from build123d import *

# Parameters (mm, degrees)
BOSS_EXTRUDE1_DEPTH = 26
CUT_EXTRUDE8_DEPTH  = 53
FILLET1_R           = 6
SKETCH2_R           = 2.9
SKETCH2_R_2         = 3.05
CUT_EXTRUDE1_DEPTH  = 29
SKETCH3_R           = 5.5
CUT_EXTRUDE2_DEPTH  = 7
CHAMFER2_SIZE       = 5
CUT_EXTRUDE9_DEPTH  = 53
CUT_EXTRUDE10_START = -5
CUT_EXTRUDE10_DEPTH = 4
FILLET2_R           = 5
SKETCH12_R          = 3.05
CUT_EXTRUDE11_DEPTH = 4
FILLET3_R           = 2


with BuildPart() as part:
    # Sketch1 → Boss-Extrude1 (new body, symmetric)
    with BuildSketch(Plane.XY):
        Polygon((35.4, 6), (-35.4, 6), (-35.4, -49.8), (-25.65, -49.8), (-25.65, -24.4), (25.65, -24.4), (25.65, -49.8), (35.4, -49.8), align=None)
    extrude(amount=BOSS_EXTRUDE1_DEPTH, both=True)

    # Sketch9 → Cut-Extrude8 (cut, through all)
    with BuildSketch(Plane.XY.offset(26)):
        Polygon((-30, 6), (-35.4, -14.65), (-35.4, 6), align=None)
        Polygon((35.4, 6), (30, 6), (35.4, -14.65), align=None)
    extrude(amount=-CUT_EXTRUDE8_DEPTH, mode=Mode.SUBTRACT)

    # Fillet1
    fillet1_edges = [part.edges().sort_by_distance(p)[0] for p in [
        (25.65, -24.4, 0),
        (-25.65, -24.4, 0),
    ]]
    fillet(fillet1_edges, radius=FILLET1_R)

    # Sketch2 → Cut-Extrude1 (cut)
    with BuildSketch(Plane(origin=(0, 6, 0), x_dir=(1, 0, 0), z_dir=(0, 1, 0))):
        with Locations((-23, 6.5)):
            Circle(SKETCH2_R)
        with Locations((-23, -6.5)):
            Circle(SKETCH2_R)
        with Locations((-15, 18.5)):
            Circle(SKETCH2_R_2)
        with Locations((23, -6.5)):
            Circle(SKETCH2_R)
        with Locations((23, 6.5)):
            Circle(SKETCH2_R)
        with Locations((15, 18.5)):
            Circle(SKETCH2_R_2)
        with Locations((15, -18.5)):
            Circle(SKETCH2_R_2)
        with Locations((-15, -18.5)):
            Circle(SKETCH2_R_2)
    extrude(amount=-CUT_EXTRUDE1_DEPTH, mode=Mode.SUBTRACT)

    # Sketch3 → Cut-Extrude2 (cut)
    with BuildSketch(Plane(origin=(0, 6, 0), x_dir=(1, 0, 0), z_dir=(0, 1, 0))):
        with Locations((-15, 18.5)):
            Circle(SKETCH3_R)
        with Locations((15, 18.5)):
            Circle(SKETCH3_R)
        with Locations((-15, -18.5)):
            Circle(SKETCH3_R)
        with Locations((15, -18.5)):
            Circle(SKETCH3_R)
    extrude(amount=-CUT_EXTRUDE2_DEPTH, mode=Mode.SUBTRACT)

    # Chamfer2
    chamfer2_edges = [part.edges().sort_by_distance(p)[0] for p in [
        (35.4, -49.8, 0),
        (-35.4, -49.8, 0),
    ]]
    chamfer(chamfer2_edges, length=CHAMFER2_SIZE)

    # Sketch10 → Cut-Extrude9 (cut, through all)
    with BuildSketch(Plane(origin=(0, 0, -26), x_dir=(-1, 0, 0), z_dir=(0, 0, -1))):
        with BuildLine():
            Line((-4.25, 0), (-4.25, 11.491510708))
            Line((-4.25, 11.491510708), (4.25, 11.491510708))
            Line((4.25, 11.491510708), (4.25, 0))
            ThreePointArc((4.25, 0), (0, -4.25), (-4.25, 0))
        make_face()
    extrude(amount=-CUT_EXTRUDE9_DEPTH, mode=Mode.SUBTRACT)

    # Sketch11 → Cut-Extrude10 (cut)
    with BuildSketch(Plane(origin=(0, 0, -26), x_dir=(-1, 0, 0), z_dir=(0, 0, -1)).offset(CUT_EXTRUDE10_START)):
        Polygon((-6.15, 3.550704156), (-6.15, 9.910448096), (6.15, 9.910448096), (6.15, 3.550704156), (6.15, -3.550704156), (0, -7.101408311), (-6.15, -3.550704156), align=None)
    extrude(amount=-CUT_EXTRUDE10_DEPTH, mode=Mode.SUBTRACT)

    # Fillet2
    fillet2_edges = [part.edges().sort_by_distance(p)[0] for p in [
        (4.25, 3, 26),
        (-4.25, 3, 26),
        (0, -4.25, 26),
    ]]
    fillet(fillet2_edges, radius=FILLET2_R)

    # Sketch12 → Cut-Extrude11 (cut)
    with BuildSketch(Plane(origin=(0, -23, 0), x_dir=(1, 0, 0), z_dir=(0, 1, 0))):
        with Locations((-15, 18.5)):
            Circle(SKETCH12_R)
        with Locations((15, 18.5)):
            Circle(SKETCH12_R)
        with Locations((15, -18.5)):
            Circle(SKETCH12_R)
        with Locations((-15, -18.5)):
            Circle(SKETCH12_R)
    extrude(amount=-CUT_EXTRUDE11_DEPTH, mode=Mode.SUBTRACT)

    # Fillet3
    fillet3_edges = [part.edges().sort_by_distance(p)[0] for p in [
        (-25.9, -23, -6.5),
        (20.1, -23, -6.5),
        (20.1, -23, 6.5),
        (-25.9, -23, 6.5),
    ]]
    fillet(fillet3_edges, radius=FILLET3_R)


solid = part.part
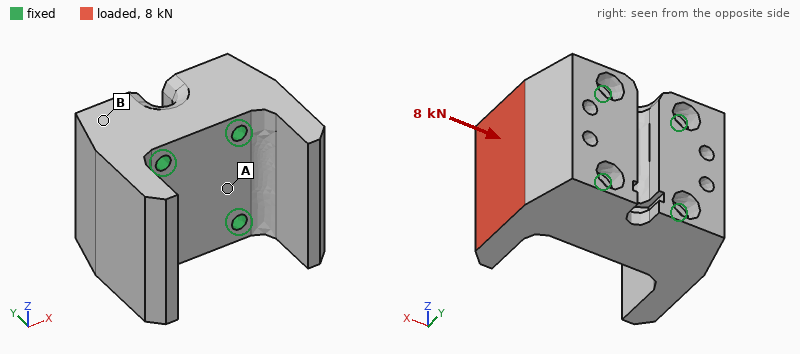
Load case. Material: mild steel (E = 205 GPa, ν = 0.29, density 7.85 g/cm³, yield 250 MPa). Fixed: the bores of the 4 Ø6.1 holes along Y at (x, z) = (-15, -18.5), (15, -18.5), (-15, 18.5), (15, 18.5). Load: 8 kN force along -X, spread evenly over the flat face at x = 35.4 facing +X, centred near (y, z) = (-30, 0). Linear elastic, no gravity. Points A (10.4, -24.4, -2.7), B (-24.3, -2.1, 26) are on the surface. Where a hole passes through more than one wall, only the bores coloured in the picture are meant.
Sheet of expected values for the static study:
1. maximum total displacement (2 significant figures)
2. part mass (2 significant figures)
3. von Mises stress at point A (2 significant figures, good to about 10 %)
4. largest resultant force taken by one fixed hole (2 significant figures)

21 µm
930 g
15 MPa
3.4 kN
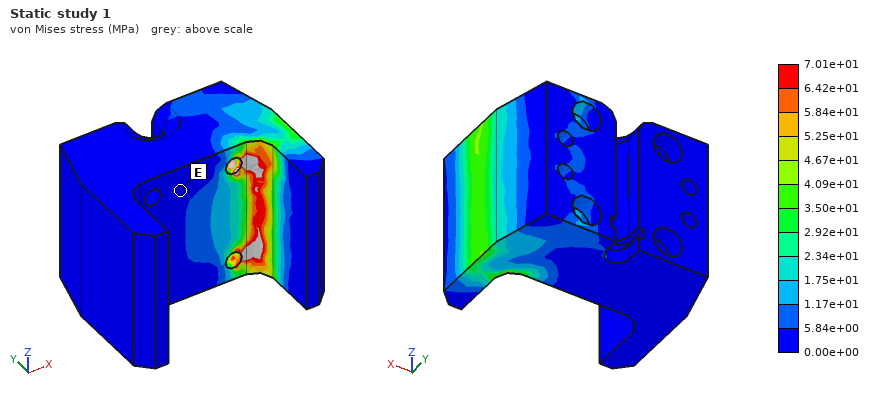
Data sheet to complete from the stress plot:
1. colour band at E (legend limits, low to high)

0.00e+00 to 5.84e+00 MPa
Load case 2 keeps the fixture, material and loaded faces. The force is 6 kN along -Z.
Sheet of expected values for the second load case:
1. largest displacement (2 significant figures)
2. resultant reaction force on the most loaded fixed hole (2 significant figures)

6.2 µm
4.5 kN
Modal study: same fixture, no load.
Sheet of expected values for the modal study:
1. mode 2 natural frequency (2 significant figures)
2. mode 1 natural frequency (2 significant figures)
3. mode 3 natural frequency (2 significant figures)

9200 Hz
9200 Hz
13 kHz
